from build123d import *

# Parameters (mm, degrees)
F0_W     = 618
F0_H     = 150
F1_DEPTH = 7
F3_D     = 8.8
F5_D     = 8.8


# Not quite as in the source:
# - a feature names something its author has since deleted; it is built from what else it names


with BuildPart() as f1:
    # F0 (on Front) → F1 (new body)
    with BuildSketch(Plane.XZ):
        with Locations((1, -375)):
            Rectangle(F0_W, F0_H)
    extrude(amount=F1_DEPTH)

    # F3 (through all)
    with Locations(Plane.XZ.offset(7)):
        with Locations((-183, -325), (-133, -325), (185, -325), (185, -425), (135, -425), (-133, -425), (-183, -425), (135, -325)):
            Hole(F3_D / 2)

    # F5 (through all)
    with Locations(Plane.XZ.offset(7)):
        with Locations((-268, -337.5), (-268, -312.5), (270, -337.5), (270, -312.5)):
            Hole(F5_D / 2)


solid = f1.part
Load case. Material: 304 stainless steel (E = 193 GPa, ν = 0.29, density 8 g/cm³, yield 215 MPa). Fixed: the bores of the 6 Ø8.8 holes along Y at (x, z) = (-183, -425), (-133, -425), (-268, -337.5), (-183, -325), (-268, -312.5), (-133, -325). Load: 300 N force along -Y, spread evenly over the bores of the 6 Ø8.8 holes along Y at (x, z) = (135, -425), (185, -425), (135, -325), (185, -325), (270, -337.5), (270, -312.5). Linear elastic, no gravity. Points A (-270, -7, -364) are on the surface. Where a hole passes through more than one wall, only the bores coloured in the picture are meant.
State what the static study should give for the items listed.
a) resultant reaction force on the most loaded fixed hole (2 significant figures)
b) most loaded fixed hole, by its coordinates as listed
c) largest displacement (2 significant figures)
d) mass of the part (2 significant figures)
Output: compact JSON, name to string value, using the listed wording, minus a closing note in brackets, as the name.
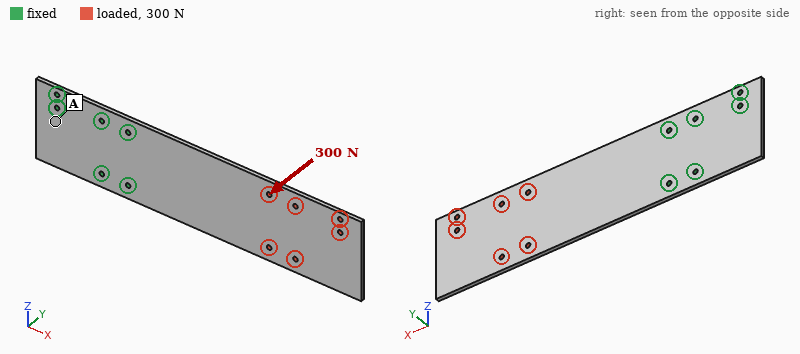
{"resultant reaction force on the most loaded fixed hole": "580 N", "most loaded fixed hole, by its coordinates as listed": "(-133, -325)", "largest displacement": "6.8 mm", "mass of the part": "5.2 kg"}
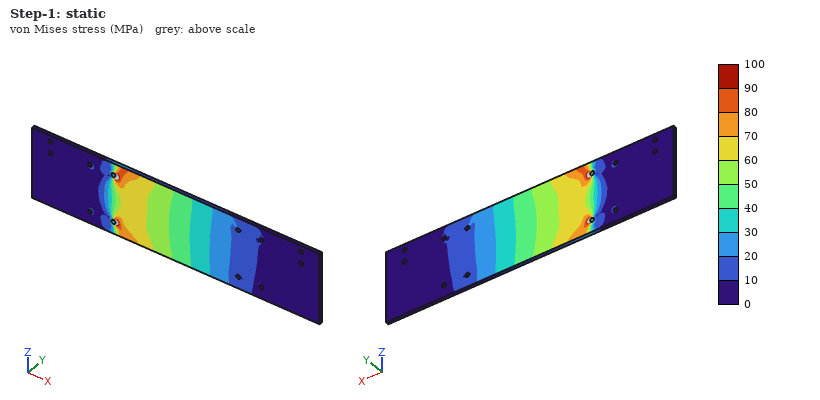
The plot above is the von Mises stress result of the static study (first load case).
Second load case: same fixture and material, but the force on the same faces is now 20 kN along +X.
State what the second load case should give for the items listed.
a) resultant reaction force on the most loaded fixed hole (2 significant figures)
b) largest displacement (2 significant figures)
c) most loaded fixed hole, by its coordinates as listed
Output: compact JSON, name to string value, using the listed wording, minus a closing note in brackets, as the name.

{"resultant reaction force on the most loaded fixed hole": "9.8 kN", "largest displacement": "0.11 mm", "most loaded fixed hole, by its coordinates as listed": "(-133, -325)"}
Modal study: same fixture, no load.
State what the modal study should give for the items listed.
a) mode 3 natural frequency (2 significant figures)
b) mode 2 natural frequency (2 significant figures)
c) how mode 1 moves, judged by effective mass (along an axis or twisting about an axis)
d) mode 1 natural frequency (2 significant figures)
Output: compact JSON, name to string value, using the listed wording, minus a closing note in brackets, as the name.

{"mode 3 natural frequency": "180 Hz", "mode 2 natural frequency": "170 Hz", "how mode 1 moves, judged by effective mass": "along Y", "mode 1 natural frequency": "28 Hz"}
